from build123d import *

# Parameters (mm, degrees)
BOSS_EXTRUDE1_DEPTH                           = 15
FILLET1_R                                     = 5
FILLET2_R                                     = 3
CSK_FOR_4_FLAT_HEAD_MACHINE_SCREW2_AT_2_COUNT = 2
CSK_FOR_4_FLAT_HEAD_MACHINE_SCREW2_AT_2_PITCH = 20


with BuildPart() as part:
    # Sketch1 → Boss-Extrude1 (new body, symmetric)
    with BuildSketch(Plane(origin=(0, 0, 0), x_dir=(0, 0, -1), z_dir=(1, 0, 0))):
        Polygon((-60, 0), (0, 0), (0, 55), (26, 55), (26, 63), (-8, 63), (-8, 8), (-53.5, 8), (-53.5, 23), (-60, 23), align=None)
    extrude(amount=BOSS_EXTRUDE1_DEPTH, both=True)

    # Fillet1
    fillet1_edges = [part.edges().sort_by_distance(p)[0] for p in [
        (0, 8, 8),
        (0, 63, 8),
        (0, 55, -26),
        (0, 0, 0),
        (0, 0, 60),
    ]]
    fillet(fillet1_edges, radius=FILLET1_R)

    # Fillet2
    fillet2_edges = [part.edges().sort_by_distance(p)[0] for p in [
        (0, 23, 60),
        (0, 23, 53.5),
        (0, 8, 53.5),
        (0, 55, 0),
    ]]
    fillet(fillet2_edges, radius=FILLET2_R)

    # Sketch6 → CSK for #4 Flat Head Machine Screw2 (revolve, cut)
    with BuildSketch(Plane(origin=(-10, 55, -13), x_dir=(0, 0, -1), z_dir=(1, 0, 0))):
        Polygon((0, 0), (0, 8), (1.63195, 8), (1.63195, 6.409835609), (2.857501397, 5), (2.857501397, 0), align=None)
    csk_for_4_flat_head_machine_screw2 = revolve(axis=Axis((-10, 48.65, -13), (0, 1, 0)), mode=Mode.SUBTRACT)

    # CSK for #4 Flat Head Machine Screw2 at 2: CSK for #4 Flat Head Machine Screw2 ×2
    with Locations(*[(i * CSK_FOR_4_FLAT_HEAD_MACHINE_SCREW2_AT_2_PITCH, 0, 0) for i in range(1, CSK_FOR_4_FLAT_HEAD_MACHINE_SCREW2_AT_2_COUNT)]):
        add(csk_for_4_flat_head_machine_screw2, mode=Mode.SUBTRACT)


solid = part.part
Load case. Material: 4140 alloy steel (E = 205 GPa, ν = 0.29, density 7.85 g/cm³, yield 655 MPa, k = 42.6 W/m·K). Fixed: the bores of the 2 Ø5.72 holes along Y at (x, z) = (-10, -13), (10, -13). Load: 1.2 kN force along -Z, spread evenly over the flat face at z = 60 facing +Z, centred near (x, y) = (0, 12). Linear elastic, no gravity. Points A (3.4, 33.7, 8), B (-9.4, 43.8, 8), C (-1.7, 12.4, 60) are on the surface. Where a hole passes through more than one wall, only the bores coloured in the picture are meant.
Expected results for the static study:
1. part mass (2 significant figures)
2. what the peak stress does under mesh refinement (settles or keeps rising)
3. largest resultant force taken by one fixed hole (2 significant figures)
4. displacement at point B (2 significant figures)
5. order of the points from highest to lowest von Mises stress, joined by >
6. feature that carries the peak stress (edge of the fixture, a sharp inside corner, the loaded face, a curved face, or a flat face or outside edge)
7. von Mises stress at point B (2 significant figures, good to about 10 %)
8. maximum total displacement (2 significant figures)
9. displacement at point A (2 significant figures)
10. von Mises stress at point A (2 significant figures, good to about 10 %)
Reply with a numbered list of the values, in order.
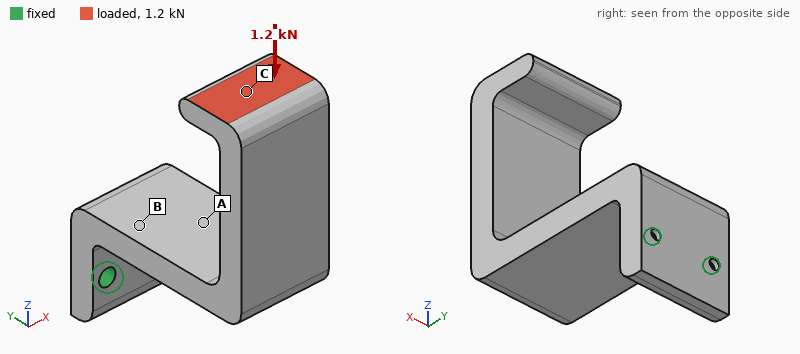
1. 280 g
2. keeps rising
3. 760 N
4. 0.085 mm
5. B > A > C
6. edge of the fixture
7. 120 MPa
8. 0.54 mm
9. 0.14 mm
10. 76 MPa
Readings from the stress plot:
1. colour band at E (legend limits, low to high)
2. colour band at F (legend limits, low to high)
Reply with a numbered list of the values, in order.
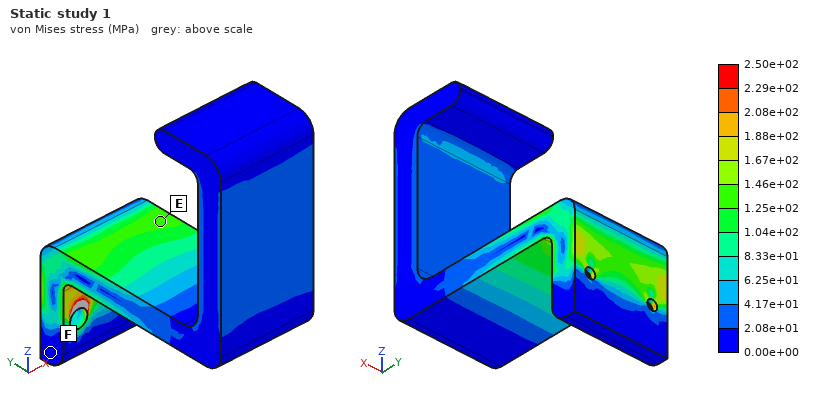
1. 1.25e+02 to 1.46e+02 MPa
2. 0.00e+00 to 2.08e+01 MPa
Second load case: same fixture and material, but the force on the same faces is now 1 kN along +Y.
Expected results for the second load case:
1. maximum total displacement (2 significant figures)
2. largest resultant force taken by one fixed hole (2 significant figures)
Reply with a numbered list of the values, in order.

1. 1.1 mm
2. 720 N
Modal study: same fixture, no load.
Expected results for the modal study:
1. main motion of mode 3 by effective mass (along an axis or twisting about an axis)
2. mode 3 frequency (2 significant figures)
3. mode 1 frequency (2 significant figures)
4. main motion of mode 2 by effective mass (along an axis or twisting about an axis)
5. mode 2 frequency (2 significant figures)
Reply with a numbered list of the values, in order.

1. along Z
2. 1600 Hz
3. 510 Hz
4. along X
5. 940 Hz
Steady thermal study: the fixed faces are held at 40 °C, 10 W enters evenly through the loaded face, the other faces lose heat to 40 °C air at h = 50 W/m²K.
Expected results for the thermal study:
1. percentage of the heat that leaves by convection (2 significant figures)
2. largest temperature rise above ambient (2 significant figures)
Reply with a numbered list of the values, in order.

1. 83 %
2. 45 K
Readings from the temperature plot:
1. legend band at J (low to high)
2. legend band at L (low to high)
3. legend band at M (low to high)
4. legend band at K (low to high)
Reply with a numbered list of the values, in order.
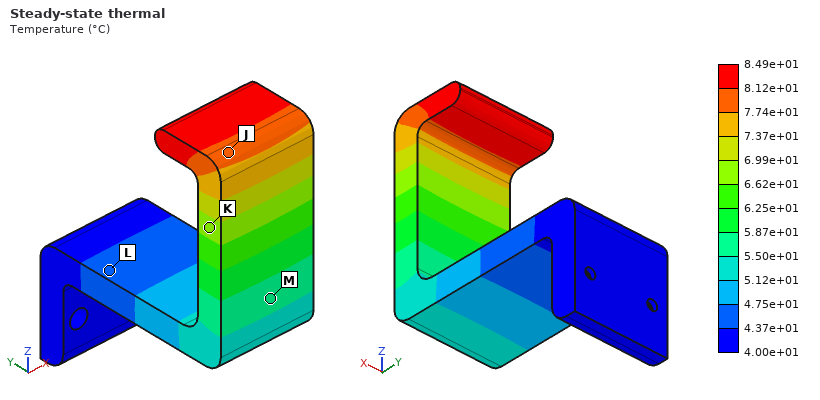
1. 7.74e+01 to 8.12e+01 °C
2. 4.37e+01 to 4.75e+01 °C
3. 5.50e+01 to 5.87e+01 °C
4. 6.62e+01 to 6.99e+01 °C
